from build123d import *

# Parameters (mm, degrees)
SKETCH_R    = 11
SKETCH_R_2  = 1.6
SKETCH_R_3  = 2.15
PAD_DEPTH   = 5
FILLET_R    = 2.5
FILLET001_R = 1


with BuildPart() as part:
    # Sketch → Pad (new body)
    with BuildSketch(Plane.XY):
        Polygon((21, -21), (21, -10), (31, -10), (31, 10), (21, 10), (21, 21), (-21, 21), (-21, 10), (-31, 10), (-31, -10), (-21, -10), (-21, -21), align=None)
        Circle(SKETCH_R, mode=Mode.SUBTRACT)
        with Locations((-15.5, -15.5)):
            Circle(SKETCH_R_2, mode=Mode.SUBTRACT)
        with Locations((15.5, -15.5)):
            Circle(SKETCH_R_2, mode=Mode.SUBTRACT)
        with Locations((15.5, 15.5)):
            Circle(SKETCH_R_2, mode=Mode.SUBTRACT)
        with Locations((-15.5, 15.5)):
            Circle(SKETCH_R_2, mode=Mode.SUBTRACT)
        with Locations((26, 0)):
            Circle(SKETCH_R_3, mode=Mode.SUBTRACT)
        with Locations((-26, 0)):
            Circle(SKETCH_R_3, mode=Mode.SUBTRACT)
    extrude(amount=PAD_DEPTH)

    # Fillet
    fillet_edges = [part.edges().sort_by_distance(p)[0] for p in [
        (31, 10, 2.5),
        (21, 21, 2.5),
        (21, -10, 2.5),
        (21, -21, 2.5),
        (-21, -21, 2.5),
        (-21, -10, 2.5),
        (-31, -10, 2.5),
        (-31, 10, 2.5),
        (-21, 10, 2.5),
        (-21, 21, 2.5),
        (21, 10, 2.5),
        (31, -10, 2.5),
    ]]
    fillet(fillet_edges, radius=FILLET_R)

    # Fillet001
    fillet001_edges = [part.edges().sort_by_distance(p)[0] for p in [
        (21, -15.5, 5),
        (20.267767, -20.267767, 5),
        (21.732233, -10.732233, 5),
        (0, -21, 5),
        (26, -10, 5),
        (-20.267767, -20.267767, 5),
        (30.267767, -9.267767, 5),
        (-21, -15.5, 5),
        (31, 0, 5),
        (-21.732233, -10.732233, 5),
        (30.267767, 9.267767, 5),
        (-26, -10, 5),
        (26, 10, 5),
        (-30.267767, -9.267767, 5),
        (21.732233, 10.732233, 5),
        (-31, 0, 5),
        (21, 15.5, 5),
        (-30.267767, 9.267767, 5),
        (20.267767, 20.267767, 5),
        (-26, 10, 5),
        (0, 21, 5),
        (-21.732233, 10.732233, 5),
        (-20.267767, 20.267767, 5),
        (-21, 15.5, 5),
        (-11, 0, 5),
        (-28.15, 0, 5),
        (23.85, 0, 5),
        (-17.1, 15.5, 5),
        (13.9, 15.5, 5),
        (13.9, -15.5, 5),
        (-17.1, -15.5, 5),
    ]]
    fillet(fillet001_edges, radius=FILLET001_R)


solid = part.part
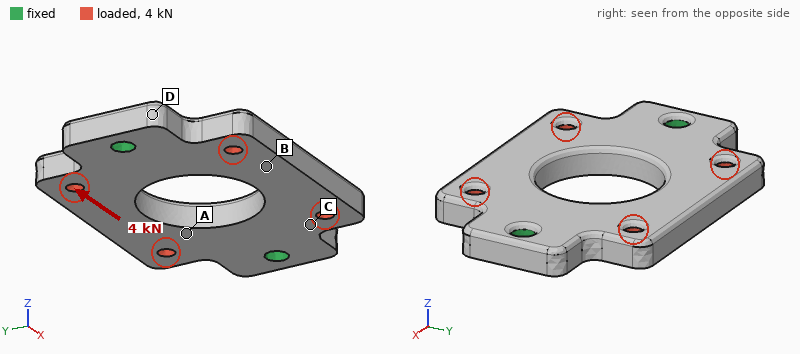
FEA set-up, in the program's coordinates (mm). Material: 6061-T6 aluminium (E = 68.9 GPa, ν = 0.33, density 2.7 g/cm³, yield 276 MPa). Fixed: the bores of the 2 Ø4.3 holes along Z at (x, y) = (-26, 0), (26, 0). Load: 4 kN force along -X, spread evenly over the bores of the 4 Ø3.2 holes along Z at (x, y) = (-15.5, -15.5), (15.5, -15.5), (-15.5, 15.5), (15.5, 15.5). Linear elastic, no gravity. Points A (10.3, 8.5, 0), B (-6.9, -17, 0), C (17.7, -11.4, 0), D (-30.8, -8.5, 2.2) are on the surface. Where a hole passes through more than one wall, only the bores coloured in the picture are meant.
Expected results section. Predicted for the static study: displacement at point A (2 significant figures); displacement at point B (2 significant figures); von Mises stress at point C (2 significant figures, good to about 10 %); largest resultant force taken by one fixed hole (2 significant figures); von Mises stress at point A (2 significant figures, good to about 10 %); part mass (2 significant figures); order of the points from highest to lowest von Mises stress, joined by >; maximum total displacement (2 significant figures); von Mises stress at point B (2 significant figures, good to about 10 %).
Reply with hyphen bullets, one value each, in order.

- 7.7 µm
- 10 µm
- 32 MPa
- 2.0 kN
- 21 MPa
- 23 g
- C > A > B > D
- 13 µm
- 14 MPa
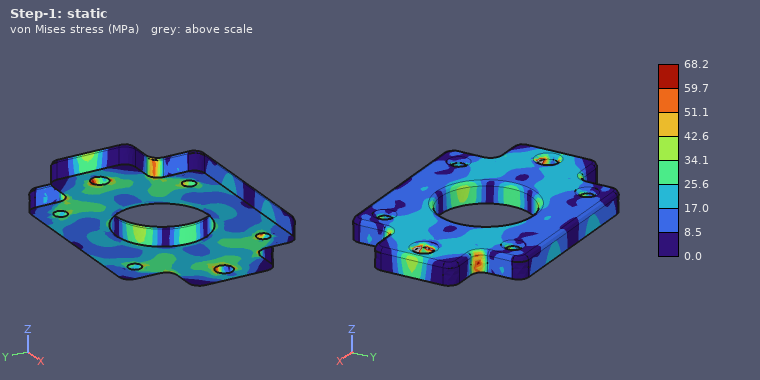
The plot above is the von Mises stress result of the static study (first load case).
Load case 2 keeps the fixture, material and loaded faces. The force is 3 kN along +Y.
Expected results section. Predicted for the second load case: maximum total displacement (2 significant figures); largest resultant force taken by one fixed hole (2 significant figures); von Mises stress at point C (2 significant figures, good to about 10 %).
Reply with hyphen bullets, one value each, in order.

- 14 µm
- 1.5 kN
- 23 MPa
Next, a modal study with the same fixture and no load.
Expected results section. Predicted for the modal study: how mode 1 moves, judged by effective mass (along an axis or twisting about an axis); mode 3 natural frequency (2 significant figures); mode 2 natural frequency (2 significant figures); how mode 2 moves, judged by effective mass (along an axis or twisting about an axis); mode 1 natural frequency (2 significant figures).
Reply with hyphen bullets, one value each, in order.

- twisting about X
- 12 kHz
- 6000 Hz
- along Z
- 5000 Hz
